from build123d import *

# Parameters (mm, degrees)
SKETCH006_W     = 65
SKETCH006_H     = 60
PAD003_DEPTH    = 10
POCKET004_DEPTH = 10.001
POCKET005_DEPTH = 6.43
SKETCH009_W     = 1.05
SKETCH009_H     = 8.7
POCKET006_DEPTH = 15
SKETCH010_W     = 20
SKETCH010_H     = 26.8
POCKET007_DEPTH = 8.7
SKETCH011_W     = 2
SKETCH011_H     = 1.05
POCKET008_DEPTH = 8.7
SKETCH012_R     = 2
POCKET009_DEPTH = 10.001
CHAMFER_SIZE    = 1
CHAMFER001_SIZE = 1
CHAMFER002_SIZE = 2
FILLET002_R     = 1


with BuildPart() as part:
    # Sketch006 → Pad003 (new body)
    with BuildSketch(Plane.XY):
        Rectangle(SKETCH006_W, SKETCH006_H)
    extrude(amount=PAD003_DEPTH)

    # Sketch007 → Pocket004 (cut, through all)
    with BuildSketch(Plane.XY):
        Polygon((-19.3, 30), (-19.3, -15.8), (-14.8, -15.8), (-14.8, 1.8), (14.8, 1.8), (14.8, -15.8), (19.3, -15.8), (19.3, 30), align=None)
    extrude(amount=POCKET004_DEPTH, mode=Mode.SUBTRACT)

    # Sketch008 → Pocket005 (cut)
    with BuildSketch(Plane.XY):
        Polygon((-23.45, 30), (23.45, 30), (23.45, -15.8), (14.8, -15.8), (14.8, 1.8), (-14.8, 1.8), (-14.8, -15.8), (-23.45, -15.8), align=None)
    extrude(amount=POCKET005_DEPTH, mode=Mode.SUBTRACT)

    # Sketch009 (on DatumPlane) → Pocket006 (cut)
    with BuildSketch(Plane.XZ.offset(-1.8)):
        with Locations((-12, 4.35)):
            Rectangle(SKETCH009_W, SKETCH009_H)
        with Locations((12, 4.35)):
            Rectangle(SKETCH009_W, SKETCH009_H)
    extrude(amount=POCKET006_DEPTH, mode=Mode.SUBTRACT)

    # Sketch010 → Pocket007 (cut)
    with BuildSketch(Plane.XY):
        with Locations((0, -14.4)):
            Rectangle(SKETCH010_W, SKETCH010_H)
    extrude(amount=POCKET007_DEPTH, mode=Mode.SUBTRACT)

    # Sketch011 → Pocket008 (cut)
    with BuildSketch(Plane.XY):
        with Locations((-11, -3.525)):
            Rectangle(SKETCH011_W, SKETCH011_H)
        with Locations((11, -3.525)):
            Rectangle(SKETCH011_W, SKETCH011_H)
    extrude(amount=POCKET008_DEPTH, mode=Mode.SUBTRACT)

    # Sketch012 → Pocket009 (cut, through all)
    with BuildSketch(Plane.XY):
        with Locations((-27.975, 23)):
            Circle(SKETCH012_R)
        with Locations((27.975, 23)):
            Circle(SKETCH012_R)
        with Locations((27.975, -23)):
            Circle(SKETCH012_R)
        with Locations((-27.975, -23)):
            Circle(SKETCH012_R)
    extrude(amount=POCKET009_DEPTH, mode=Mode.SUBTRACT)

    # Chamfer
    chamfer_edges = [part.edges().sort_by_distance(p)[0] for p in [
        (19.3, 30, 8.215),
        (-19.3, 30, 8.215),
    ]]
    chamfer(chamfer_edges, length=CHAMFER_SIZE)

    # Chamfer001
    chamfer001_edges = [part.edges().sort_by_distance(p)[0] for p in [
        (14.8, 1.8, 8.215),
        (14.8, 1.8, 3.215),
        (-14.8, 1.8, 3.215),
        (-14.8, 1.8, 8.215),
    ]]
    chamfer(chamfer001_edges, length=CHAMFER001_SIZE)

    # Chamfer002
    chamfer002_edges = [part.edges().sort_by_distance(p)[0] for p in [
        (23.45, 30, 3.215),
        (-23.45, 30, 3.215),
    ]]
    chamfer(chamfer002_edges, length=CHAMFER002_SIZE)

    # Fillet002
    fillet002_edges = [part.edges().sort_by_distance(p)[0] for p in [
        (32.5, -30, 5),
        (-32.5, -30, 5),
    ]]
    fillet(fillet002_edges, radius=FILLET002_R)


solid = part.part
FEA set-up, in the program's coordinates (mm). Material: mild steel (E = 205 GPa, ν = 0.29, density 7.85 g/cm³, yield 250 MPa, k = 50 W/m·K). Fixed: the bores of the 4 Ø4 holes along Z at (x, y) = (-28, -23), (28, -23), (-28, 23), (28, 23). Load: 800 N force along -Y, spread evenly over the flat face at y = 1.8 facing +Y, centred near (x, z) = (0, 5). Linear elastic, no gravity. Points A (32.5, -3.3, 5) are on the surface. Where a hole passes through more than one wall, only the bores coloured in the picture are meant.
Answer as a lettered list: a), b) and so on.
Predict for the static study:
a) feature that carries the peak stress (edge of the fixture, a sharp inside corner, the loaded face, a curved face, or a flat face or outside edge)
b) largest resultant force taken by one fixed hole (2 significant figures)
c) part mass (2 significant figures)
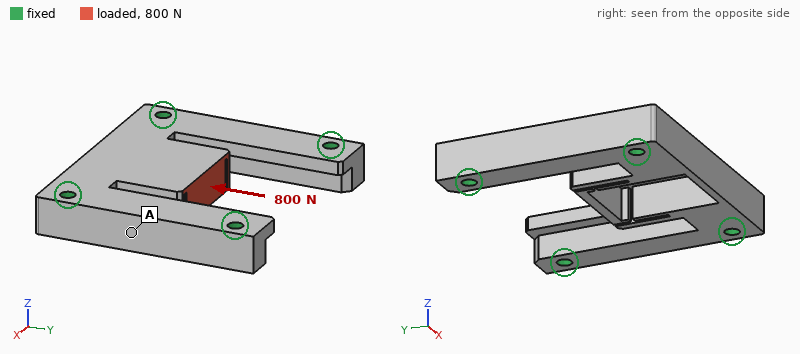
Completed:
a) the loaded face
b) 320 N
c) 150 g
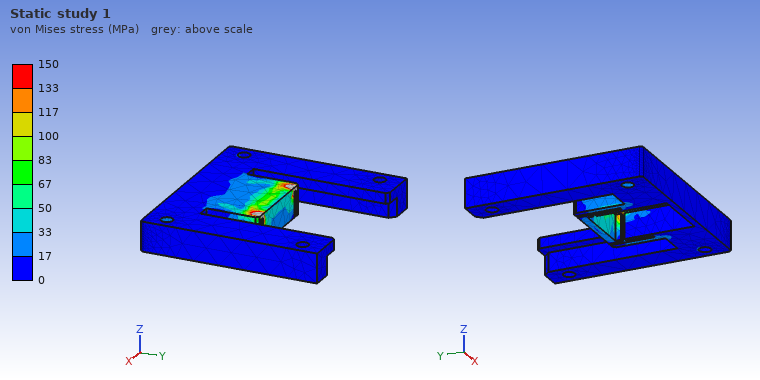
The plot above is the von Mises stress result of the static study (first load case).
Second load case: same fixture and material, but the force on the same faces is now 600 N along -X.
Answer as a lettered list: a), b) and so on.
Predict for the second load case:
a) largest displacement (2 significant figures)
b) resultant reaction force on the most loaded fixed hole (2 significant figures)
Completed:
a) 21 µm
b) 430 N
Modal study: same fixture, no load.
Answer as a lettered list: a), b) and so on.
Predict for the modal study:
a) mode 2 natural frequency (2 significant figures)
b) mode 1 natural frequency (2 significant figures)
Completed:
a) 8800 Hz
b) 7100 Hz
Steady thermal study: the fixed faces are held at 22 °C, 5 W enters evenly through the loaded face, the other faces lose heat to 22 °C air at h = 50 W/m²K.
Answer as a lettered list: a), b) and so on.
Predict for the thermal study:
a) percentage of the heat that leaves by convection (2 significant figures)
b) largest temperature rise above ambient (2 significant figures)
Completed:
a) 41 %
b) 29 K
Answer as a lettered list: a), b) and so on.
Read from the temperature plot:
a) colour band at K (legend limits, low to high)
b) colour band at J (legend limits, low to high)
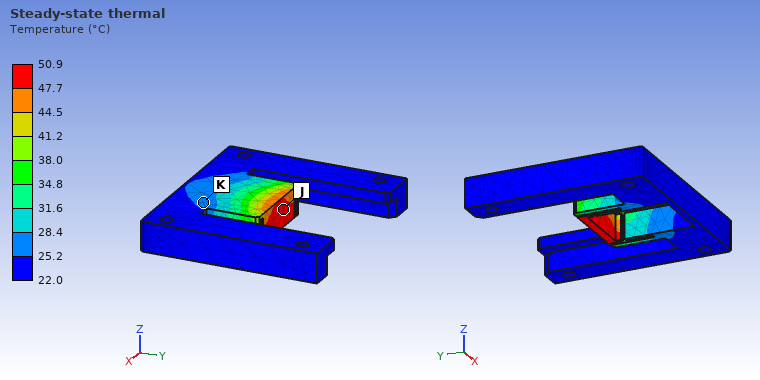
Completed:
a) 25.2 to 28.4 °C
b) 47.7 to 50.9 °C
